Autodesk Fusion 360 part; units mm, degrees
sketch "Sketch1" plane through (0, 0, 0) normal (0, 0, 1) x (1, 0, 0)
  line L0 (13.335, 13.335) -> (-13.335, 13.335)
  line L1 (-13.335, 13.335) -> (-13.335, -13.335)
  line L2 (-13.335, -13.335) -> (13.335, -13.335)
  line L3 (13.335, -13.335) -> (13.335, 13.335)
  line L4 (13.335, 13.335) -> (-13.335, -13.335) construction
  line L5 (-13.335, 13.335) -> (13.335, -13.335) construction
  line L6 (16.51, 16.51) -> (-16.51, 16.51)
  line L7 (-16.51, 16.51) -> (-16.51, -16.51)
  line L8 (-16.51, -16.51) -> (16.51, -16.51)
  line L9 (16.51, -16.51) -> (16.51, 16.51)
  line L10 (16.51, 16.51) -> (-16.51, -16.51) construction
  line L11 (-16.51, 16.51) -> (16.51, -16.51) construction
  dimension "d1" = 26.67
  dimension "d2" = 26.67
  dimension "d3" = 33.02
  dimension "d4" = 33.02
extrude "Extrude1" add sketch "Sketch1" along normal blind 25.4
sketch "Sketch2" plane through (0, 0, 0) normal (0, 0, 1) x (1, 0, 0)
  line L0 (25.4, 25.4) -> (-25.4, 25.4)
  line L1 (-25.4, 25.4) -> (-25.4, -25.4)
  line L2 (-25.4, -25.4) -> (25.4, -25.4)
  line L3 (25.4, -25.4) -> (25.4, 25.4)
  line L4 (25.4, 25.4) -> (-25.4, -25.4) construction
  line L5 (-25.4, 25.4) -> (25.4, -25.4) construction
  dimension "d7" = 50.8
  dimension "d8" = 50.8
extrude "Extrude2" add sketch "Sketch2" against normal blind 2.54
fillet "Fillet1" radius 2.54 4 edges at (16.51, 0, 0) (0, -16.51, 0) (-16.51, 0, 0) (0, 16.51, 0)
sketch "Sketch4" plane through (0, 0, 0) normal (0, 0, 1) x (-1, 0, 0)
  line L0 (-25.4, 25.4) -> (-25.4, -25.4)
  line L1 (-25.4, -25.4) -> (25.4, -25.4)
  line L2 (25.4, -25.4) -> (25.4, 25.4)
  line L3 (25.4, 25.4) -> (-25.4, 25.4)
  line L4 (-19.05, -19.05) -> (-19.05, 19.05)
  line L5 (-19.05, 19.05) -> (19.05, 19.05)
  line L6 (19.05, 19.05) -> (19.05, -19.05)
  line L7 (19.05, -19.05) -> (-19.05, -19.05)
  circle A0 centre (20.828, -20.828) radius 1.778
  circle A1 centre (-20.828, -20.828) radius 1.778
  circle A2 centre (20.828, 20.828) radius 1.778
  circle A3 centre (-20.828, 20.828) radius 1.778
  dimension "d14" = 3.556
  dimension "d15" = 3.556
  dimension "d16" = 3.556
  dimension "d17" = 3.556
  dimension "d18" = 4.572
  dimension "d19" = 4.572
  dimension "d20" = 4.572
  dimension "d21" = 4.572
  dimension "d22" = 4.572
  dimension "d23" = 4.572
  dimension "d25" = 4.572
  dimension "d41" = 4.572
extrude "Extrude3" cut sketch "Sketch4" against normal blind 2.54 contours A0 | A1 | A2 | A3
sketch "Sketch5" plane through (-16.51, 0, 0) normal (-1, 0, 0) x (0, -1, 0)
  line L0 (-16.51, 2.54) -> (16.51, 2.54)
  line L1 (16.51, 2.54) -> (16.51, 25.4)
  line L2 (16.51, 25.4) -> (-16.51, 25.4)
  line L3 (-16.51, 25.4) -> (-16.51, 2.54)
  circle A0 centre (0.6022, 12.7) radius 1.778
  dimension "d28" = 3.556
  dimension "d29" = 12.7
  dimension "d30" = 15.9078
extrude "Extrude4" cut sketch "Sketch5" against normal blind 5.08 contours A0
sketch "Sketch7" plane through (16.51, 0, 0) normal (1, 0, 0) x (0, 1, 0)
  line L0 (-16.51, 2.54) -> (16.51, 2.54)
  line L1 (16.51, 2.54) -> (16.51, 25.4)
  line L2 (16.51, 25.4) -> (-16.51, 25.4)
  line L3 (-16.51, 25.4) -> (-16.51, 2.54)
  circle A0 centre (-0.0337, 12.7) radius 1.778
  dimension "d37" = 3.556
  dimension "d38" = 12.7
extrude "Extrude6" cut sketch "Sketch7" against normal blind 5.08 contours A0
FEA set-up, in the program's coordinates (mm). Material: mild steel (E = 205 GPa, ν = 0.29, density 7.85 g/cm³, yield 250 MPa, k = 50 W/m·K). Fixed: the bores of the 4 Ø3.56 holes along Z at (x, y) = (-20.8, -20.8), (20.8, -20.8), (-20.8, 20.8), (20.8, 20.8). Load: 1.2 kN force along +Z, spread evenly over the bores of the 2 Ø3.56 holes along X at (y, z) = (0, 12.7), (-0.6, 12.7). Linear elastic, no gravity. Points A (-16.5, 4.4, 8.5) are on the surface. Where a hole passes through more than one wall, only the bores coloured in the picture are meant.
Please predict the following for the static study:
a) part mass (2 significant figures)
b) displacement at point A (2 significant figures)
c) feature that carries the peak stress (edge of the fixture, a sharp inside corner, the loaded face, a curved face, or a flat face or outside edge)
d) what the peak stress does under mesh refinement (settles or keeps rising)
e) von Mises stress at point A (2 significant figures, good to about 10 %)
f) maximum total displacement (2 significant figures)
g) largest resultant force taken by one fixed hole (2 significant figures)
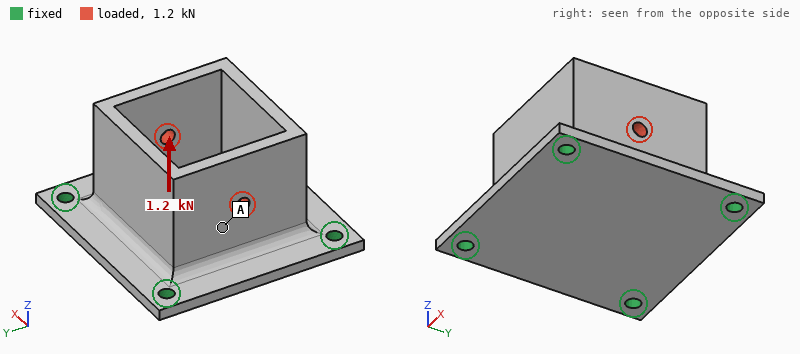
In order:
130 g
4.8 µm
edge of the fixture
keeps rising
9.5 MPa
5.2 µm
360 N
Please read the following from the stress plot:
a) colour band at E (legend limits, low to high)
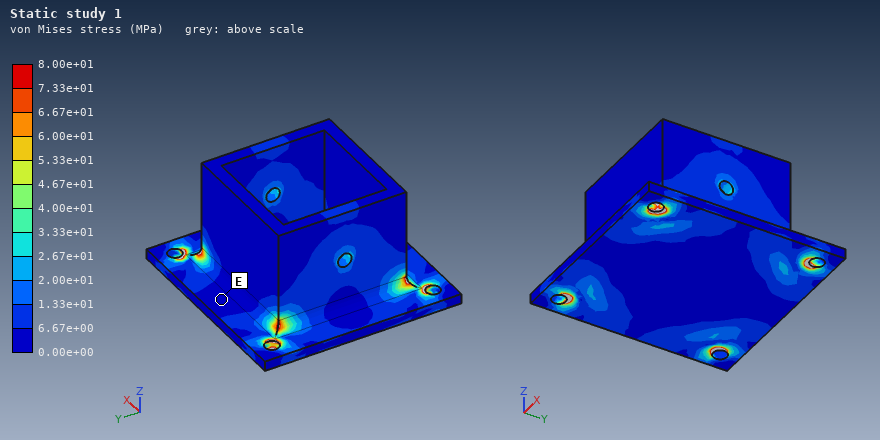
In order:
0.00e+00 to 6.67e+00 MPa
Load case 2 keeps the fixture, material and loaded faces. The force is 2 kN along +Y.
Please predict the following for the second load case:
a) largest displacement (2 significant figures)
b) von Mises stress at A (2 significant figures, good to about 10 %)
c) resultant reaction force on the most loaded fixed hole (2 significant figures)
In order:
10 µm
19 MPa
660 N
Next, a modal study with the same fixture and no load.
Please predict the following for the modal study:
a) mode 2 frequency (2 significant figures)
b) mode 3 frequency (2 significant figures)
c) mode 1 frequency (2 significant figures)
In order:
7700 Hz
7800 Hz
7700 Hz
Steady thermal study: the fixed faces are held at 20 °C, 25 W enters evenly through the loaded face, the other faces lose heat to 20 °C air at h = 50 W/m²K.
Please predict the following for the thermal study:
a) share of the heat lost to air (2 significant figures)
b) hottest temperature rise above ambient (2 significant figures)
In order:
45 %
52 K
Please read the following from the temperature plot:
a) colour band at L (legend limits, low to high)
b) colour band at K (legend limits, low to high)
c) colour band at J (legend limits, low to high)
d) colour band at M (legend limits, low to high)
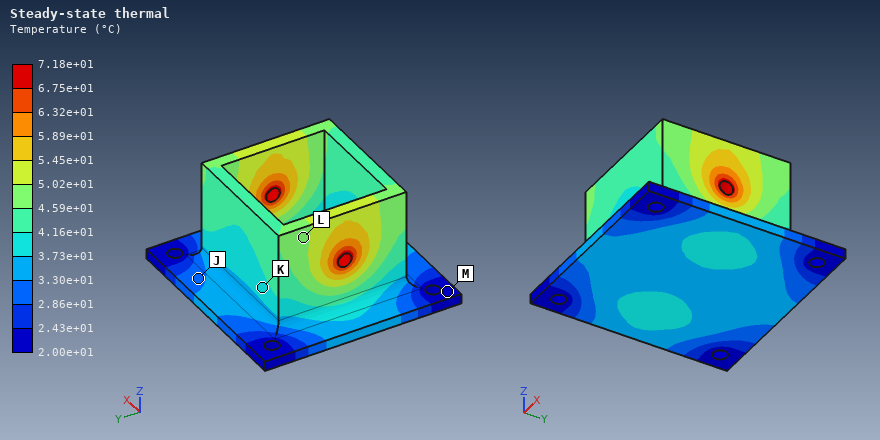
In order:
4.59e+01 to 5.02e+01 °C
3.73e+01 to 4.16e+01 °C
2.86e+01 to 3.30e+01 °C
2.00e+01 to 2.43e+01 °C
